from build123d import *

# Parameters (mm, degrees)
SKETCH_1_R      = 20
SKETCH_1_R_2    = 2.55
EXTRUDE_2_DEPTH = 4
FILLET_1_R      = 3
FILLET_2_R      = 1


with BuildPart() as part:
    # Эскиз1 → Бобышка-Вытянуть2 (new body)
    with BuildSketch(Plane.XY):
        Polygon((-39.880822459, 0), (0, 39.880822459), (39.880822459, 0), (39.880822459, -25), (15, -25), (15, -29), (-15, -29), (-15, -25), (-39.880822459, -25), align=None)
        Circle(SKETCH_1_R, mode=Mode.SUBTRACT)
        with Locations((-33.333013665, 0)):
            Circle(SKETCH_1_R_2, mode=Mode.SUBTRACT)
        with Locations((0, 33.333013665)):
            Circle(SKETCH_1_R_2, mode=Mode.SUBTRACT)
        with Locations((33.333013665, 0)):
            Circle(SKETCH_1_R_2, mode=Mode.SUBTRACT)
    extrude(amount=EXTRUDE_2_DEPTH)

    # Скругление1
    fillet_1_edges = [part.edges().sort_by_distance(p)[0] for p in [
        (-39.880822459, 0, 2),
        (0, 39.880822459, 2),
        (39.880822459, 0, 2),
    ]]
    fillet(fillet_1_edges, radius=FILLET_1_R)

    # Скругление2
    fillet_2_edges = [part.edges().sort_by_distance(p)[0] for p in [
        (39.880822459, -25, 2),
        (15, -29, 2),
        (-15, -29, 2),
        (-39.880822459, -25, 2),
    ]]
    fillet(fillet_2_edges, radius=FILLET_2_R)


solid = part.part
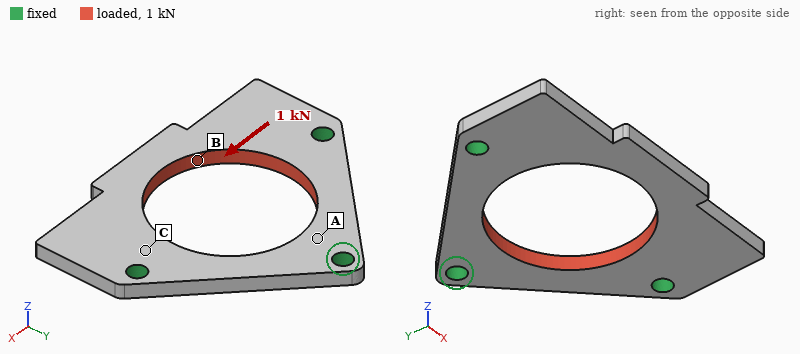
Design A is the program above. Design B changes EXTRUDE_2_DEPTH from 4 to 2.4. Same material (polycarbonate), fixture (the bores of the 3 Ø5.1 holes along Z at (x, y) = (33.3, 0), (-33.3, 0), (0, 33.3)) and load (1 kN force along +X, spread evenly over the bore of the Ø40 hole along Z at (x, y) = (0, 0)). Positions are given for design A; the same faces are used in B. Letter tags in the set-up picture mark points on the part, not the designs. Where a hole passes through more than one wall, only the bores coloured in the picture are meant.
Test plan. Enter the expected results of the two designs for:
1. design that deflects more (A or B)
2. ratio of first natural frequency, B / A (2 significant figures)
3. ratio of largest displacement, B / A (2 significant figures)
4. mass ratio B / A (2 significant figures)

B
0.62
1.7
0.60
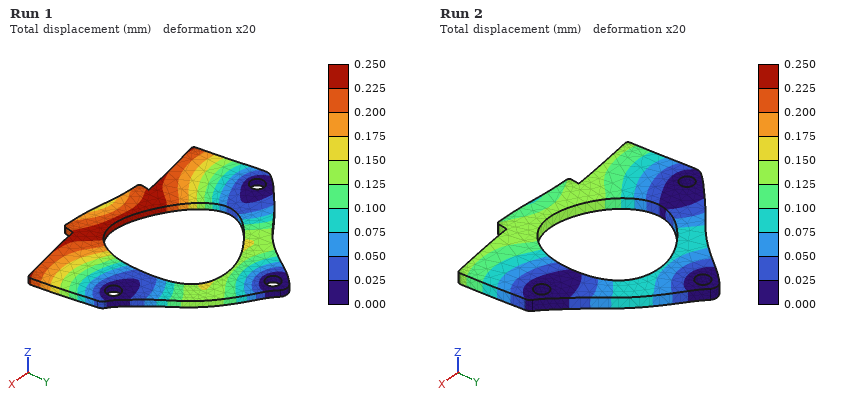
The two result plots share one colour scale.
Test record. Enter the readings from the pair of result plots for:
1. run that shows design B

Run 1
